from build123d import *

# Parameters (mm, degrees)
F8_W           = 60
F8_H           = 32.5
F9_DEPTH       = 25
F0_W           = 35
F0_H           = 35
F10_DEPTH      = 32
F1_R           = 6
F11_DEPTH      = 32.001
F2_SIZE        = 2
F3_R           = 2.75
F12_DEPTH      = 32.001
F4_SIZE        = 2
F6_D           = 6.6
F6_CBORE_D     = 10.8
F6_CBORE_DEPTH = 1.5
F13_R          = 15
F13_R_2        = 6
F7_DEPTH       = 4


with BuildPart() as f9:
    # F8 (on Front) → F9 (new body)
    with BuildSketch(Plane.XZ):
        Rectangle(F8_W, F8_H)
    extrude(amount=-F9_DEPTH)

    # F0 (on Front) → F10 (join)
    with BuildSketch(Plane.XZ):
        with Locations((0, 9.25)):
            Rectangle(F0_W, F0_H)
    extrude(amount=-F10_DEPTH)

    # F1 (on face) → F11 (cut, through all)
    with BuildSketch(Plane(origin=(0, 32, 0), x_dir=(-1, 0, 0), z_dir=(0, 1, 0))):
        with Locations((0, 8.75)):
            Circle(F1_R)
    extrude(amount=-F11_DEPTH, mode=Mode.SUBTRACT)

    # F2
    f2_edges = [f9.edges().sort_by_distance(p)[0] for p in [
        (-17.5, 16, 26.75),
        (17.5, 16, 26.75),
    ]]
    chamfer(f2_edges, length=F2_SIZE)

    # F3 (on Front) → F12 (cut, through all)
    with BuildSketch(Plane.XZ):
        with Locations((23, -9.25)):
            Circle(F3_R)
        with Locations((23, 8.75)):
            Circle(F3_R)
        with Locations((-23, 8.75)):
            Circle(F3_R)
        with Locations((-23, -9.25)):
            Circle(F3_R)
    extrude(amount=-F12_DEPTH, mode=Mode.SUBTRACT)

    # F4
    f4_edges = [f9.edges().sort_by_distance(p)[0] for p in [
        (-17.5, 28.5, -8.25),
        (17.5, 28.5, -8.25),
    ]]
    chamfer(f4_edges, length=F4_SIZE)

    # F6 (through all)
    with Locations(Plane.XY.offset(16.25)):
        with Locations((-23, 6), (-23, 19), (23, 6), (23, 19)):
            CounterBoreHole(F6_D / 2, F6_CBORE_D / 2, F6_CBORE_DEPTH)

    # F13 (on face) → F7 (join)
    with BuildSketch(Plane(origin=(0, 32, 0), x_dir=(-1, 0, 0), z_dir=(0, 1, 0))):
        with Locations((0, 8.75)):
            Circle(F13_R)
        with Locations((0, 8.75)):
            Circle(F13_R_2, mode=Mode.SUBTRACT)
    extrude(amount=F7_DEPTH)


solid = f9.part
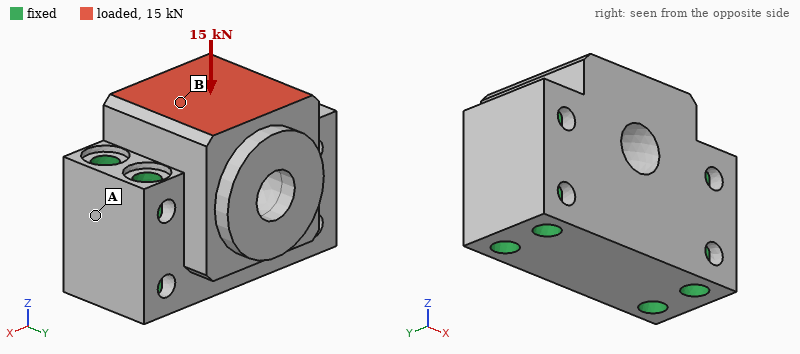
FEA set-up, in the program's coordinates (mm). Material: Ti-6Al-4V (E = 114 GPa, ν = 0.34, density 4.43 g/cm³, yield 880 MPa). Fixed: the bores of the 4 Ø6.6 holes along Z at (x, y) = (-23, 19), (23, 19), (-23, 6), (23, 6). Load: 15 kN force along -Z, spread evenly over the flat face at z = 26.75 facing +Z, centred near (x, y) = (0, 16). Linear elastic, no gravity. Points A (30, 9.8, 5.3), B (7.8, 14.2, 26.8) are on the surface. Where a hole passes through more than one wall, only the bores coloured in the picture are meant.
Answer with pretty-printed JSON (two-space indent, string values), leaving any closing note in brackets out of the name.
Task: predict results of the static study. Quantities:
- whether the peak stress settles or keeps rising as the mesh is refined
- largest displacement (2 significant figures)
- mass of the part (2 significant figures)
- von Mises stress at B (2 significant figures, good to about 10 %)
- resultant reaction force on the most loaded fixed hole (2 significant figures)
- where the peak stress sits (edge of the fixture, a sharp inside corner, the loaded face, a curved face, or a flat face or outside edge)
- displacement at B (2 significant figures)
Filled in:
{
  "whether the peak stress settles or keeps rising as the mesh is refined": "keeps rising",
  "largest displacement": "7.2 µm",
  "mass of the part": "260 g",
  "von Mises stress at B": "13 MPa",
  "resultant reaction force on the most loaded fixed hole": "4.8 kN",
  "where the peak stress sits": "edge of the fixture",
  "displacement at B": "5.3 µm"
}
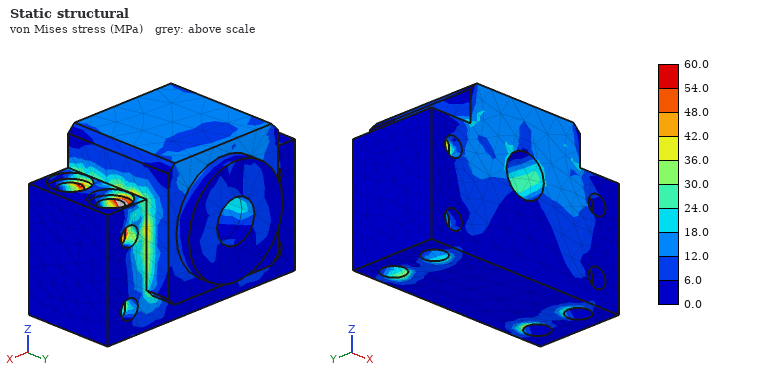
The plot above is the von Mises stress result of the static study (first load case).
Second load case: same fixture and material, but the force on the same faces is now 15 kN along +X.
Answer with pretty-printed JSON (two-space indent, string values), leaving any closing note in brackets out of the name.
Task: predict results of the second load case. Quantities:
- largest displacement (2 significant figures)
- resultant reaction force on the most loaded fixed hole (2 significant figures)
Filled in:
{
  "largest displacement": "11 µm",
  "resultant reaction force on the most loaded fixed hole": "5.6 kN"
}
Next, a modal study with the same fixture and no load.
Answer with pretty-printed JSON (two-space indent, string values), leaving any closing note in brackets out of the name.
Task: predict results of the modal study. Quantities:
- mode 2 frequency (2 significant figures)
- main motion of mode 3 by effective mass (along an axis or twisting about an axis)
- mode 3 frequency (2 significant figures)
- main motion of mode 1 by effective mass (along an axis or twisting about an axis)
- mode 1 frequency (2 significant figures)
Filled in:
{
  "mode 2 frequency": "27 kHz",
  "main motion of mode 3 by effective mass": "along X",
  "mode 3 frequency": "31 kHz",
  "main motion of mode 1 by effective mass": "along Y",
  "mode 1 frequency": "17 kHz"
}
